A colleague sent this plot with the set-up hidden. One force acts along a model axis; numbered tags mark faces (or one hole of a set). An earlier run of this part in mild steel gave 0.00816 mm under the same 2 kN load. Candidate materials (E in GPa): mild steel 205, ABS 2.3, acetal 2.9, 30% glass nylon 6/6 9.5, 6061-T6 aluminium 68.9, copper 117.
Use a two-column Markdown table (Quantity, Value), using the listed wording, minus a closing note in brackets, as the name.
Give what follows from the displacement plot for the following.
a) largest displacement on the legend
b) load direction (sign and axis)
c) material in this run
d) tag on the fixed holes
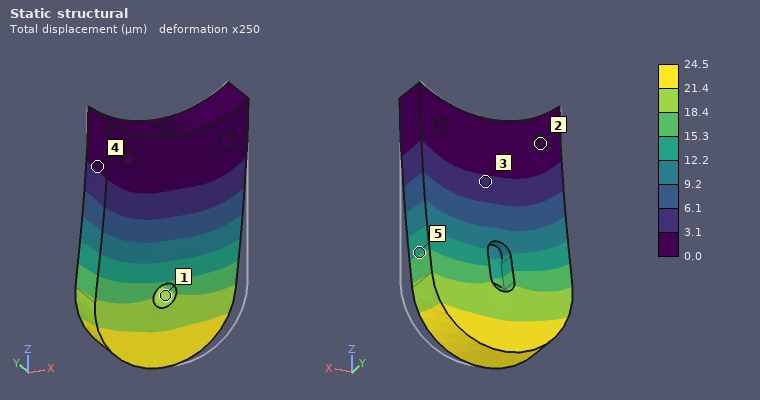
| Quantity | Value |
|---|---|
| largest displacement on the legend | 24.5 µm |
| load direction | -X |
| material in this run | 6061-T6 aluminium |
| tag on the fixed holes | 2 |
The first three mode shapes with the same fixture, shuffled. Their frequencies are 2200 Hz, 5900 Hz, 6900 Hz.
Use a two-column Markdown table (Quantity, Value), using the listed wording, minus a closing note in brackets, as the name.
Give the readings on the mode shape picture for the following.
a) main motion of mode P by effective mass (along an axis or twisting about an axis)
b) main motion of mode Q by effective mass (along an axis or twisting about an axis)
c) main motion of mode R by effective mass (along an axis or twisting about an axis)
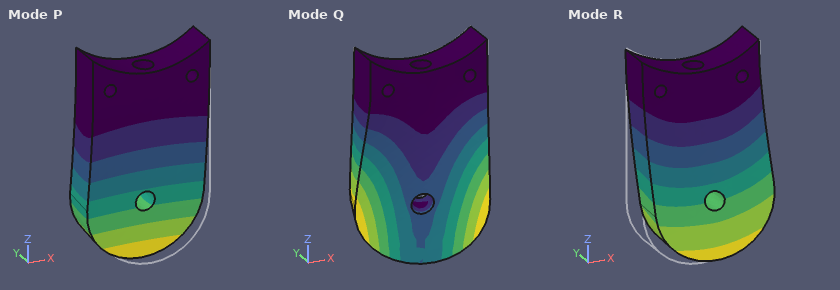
| Quantity | Value |
|---|---|
| main motion of mode P by effective mass | along Y |
| main motion of mode Q by effective mass | twisting about Z |
| main motion of mode R by effective mass | along X |
